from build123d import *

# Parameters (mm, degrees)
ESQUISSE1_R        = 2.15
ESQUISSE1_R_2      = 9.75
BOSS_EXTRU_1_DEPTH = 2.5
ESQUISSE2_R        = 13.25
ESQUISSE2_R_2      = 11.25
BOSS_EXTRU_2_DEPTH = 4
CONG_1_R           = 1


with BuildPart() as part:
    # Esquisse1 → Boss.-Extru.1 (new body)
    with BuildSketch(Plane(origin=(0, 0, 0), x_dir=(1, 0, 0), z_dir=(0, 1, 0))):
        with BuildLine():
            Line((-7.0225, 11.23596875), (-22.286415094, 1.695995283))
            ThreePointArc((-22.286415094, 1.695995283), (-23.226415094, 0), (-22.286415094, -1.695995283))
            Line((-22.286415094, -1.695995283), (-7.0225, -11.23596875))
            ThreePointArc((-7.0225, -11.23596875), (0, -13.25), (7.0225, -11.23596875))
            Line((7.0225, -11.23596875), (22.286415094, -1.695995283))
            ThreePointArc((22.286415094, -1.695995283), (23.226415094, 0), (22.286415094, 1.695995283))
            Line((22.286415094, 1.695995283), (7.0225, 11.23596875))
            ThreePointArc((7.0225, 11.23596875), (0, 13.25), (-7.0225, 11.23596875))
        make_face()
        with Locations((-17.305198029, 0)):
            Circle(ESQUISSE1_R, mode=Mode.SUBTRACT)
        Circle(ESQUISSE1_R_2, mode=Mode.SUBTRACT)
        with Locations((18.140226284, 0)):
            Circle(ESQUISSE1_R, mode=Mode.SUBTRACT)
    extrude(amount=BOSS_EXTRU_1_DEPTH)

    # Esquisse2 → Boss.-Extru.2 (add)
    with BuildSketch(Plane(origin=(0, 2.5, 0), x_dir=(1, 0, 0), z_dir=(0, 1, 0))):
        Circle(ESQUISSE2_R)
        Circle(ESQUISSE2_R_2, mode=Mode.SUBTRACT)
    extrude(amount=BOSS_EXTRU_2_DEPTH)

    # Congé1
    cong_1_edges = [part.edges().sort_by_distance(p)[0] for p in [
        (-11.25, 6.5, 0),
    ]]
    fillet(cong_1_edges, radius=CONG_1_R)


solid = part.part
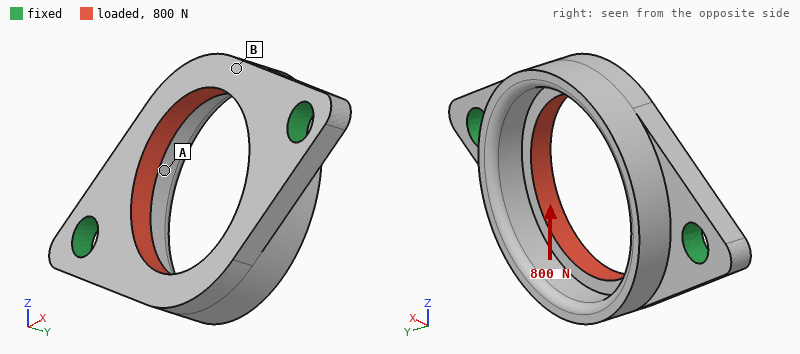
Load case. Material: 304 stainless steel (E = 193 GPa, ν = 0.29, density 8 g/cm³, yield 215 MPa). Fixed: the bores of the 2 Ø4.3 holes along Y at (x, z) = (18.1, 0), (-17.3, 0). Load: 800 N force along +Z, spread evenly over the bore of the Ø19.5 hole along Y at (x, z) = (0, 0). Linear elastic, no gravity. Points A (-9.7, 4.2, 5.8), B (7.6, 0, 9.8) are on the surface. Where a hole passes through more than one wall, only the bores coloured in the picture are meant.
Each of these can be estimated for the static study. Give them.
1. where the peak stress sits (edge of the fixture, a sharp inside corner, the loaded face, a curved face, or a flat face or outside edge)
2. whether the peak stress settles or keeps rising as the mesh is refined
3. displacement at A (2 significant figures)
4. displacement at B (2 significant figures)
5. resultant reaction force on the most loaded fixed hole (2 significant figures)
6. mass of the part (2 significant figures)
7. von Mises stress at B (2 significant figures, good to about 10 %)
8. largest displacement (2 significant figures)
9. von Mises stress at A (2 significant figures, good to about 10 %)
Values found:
edge of the fixture
keeps rising
1.2 µm
2.5 µm
400 N
13 g
22 MPa
2.9 µm
6.8 MPa
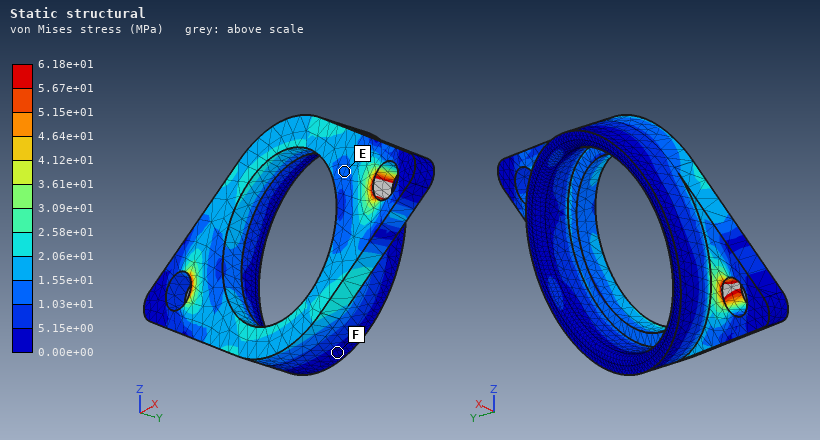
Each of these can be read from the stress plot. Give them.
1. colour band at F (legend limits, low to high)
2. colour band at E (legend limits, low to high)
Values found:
0.00e+00 to 5.15e+00 MPa
1.03e+01 to 1.55e+01 MPa
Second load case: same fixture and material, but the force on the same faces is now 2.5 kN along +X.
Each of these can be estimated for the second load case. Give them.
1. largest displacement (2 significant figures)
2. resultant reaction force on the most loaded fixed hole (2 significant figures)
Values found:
7.1 µm
1.3 kN
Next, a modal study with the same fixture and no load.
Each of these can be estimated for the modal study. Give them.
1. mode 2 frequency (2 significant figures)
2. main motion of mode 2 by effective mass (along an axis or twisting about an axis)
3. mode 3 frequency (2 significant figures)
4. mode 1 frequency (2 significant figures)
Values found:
10 kHz
along Y
21 kHz
7900 Hz
